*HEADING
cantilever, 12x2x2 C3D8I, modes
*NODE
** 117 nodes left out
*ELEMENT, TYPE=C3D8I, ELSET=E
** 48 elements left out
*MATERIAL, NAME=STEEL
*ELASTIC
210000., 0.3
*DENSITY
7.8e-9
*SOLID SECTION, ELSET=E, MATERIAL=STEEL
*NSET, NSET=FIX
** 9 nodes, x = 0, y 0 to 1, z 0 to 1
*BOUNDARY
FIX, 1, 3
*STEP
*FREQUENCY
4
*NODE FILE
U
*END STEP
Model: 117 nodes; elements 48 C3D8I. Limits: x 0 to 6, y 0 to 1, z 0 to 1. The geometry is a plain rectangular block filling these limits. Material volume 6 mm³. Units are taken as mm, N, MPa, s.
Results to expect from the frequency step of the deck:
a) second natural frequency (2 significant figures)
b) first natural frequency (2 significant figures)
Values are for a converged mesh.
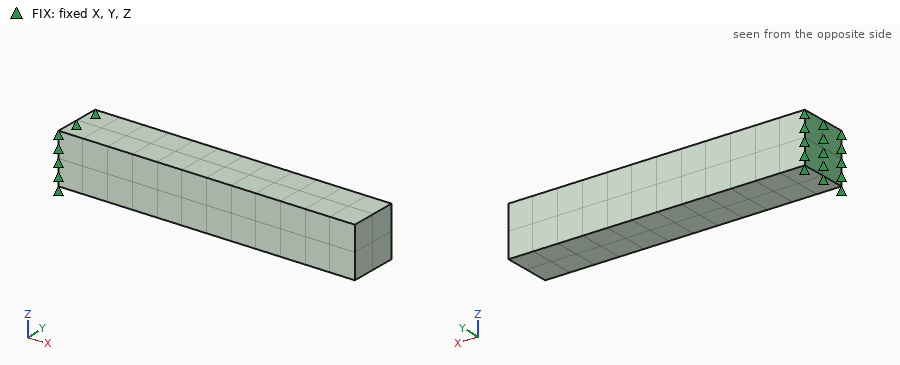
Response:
23000 Hz
23000 Hz
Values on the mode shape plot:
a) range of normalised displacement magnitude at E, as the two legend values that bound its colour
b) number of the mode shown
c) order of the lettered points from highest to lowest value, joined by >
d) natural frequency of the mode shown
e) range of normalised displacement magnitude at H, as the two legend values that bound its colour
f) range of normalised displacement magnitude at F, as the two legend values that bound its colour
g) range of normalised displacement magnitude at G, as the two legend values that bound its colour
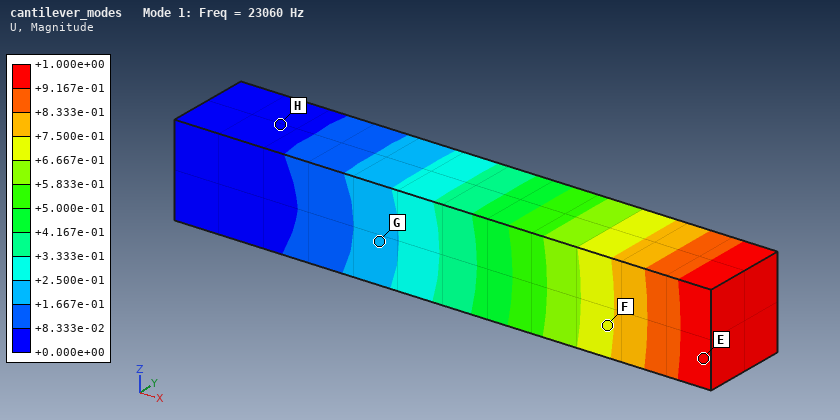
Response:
+9.167e-01 to +1.000e+00
1
E > F > G > H
23060 Hz
+0.000e+00 to +8.333e-02
+6.667e-01 to +7.500e-01
+1.667e-01 to +2.500e-01
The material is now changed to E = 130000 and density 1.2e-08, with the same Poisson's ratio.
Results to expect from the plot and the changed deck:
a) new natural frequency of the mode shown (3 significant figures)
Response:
14600 Hz
